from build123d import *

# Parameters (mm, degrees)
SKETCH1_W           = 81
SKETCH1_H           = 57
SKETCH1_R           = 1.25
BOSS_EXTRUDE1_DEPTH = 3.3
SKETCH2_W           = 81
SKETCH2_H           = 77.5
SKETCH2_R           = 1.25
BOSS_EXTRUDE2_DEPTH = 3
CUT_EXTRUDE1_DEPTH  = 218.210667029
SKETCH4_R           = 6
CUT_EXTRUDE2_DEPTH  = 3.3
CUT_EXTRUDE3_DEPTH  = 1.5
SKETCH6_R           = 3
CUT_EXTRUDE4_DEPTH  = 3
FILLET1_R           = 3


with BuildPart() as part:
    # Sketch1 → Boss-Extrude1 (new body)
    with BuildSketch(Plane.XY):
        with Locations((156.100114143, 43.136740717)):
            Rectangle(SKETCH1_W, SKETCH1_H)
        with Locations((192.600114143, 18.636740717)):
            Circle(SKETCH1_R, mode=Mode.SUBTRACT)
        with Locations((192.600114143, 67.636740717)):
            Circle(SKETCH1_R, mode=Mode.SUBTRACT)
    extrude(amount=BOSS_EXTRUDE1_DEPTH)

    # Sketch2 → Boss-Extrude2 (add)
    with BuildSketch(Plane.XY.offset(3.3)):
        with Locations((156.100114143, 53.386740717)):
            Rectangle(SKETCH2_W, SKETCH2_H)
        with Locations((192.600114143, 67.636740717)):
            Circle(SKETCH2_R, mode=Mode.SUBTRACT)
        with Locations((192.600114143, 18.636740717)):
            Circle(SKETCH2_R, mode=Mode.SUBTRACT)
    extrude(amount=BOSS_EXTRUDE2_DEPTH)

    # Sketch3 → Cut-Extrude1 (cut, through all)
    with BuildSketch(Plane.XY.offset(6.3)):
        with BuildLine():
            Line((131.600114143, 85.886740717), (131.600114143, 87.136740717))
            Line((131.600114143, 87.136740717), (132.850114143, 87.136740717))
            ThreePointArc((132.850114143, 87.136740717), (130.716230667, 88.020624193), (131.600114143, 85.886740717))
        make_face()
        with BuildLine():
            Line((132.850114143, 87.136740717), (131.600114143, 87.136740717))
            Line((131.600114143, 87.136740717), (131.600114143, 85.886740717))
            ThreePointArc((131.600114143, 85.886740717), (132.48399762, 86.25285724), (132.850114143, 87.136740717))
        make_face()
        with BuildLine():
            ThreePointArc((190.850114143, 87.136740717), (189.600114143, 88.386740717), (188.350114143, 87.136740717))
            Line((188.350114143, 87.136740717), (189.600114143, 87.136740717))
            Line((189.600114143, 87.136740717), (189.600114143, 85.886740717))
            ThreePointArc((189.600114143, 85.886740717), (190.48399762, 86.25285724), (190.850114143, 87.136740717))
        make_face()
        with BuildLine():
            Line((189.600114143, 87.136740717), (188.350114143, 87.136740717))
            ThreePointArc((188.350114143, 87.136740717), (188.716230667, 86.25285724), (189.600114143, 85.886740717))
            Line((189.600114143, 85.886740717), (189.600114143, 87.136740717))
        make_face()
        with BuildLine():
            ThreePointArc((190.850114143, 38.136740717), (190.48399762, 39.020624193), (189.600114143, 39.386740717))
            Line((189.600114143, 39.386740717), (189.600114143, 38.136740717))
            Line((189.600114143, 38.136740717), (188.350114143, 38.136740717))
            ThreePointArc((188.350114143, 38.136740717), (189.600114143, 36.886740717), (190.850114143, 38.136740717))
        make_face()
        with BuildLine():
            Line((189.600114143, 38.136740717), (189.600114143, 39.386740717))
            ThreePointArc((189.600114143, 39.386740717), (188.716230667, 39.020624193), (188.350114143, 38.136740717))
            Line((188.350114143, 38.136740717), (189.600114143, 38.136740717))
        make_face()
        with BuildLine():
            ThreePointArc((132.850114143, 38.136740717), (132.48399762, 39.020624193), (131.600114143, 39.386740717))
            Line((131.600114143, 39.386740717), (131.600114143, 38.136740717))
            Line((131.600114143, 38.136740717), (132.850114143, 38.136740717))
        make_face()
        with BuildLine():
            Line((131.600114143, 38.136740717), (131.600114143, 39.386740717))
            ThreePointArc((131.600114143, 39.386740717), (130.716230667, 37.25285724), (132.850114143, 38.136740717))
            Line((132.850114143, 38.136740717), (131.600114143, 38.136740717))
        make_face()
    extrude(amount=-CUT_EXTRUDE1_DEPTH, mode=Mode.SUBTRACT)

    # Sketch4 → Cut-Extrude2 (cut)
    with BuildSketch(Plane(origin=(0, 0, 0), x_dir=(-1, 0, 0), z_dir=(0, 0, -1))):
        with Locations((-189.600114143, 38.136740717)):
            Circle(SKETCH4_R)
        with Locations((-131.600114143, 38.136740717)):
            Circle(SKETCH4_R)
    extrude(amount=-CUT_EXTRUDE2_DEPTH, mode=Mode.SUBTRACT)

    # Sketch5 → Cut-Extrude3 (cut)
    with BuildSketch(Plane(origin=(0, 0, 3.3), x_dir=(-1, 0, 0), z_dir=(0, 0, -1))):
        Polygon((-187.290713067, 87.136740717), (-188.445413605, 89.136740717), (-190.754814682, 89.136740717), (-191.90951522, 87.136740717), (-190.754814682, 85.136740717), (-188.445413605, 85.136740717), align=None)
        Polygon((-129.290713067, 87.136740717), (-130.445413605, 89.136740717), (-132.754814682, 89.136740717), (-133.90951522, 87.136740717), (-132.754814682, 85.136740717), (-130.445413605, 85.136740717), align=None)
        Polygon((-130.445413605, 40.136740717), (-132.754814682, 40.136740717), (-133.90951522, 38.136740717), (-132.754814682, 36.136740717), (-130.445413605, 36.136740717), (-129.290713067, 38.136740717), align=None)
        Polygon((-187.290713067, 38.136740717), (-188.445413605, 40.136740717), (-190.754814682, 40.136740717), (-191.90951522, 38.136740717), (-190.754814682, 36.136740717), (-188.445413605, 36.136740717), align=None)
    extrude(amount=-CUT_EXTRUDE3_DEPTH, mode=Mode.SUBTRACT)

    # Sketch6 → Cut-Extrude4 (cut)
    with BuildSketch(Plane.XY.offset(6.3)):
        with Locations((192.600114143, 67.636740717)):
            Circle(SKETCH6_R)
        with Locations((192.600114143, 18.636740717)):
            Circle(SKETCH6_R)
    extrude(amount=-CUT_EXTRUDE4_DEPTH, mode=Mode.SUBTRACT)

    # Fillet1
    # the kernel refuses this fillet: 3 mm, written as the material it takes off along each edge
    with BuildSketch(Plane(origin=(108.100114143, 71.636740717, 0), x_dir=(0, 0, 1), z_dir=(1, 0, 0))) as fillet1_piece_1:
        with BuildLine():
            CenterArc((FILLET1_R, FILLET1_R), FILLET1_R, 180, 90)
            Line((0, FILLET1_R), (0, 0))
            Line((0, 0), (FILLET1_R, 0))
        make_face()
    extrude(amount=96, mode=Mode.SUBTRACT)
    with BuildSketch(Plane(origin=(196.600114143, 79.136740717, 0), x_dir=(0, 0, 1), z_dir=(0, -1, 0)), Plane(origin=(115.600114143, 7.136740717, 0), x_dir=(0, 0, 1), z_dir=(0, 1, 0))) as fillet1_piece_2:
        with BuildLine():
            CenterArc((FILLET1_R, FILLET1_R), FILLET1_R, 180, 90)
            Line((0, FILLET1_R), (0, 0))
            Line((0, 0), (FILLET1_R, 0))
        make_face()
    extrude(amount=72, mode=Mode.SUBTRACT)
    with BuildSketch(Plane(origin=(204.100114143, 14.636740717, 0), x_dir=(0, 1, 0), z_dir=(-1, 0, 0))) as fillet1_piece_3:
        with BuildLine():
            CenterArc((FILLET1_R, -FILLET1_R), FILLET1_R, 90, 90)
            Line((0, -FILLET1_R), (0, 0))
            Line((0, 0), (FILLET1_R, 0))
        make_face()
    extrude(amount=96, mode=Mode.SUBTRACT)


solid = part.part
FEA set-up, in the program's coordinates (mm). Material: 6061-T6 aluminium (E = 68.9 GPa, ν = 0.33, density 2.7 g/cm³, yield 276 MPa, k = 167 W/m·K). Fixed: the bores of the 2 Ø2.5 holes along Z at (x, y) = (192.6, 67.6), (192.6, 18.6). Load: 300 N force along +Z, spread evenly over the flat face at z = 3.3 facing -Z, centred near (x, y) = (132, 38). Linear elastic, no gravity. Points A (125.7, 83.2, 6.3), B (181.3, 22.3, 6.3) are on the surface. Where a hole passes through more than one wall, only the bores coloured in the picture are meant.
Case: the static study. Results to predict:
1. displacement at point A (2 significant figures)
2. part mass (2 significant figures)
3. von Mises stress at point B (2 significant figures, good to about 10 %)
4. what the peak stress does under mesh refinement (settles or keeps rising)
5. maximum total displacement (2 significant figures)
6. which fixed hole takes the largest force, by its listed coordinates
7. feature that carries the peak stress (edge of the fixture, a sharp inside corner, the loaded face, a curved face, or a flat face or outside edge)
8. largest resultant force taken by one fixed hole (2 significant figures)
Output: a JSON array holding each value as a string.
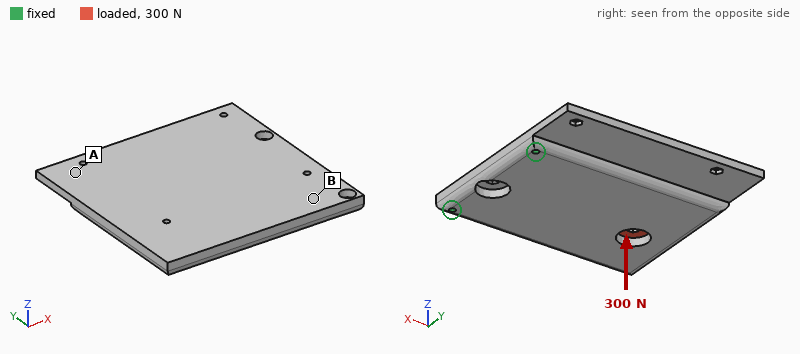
["0.82 mm", "88 g", "48 MPa", "keeps rising", "1.0 mm", "(192.6, 18.6)", "edge of the fixture", "200 N"]
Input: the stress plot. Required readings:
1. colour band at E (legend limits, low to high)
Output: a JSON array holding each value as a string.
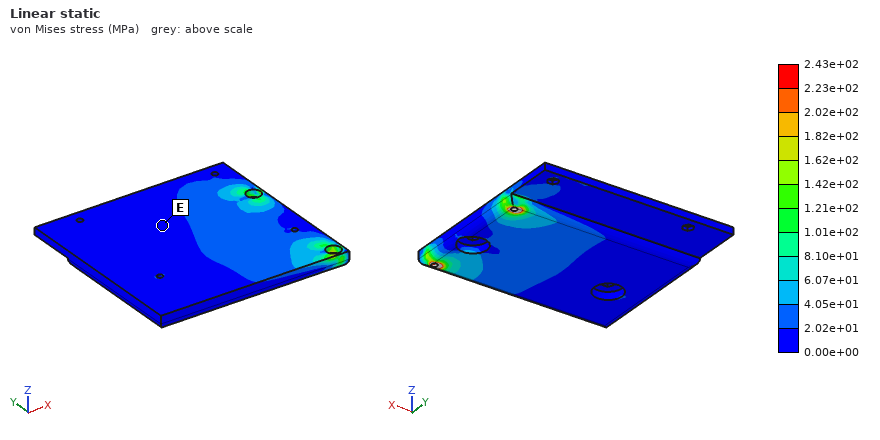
["0.00e+00 to 2.02e+01 MPa"]
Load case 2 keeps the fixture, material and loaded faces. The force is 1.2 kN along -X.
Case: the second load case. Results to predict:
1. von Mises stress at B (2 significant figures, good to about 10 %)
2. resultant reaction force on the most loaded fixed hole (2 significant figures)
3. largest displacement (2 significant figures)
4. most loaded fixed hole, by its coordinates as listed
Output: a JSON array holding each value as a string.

["6.3 MPa", "740 N", "68 µm", "(192.6, 18.6)"]
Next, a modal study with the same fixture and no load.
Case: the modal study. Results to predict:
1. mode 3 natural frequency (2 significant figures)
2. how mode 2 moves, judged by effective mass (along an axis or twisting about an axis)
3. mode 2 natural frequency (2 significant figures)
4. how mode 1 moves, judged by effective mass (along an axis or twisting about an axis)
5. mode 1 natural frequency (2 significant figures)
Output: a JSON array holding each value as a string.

["3600 Hz", "twisting about X", "1700 Hz", "along Z", "480 Hz"]
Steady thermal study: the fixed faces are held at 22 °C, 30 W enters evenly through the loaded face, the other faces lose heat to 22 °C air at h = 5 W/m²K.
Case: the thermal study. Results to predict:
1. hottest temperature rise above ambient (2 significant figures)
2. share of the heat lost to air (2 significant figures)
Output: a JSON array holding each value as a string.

["46 K", "5.6 %"]
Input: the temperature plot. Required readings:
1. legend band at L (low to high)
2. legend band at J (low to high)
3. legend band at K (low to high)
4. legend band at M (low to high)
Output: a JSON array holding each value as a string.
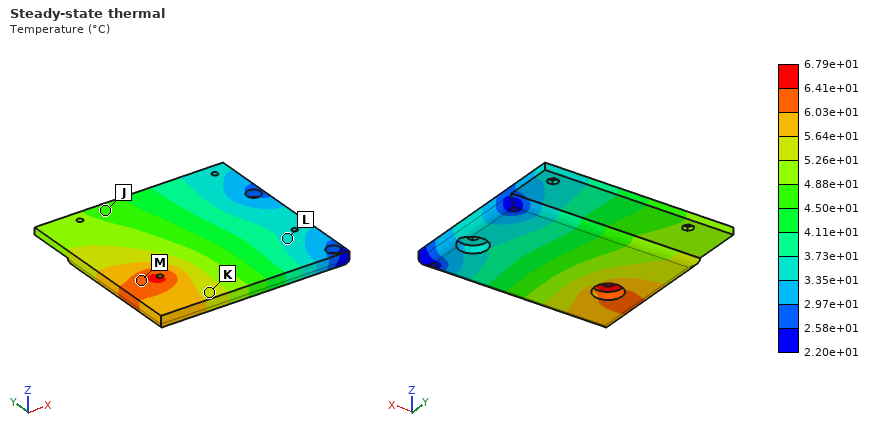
["3.35e+01 to 3.73e+01 °C", "4.50e+01 to 4.88e+01 °C", "5.26e+01 to 5.64e+01 °C", "6.03e+01 to 6.41e+01 °C"]
